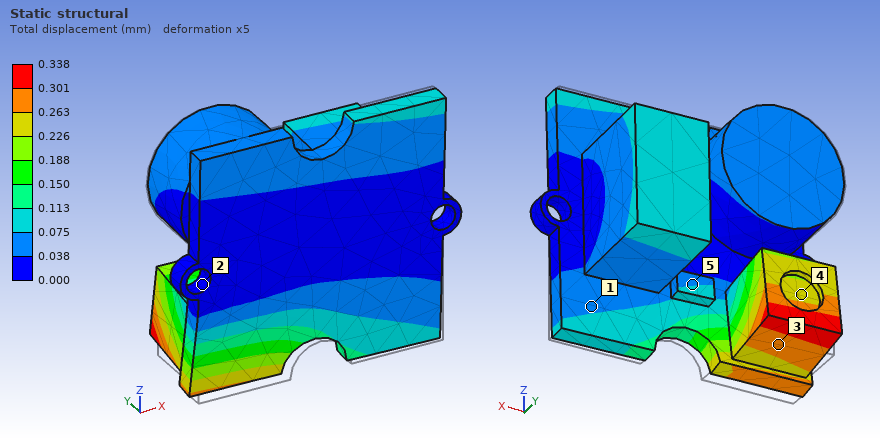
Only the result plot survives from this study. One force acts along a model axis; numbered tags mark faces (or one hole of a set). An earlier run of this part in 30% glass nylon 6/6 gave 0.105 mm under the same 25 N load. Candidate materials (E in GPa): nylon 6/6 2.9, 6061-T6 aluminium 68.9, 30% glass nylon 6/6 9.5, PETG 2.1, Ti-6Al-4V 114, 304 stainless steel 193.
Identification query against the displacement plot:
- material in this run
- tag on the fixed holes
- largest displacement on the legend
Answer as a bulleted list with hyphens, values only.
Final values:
- nylon 6/6
- 2
- 0.338 mm
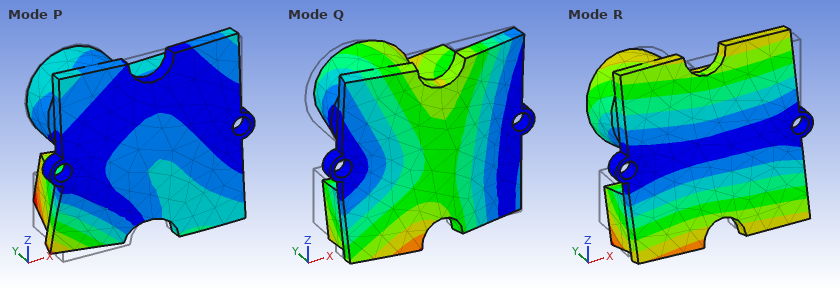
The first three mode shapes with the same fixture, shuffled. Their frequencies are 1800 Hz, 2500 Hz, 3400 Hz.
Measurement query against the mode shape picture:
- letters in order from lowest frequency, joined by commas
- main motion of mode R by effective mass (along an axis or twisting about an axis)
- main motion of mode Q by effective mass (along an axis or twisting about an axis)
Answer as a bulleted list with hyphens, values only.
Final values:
- R, Q, P
- along Z
- along Y
